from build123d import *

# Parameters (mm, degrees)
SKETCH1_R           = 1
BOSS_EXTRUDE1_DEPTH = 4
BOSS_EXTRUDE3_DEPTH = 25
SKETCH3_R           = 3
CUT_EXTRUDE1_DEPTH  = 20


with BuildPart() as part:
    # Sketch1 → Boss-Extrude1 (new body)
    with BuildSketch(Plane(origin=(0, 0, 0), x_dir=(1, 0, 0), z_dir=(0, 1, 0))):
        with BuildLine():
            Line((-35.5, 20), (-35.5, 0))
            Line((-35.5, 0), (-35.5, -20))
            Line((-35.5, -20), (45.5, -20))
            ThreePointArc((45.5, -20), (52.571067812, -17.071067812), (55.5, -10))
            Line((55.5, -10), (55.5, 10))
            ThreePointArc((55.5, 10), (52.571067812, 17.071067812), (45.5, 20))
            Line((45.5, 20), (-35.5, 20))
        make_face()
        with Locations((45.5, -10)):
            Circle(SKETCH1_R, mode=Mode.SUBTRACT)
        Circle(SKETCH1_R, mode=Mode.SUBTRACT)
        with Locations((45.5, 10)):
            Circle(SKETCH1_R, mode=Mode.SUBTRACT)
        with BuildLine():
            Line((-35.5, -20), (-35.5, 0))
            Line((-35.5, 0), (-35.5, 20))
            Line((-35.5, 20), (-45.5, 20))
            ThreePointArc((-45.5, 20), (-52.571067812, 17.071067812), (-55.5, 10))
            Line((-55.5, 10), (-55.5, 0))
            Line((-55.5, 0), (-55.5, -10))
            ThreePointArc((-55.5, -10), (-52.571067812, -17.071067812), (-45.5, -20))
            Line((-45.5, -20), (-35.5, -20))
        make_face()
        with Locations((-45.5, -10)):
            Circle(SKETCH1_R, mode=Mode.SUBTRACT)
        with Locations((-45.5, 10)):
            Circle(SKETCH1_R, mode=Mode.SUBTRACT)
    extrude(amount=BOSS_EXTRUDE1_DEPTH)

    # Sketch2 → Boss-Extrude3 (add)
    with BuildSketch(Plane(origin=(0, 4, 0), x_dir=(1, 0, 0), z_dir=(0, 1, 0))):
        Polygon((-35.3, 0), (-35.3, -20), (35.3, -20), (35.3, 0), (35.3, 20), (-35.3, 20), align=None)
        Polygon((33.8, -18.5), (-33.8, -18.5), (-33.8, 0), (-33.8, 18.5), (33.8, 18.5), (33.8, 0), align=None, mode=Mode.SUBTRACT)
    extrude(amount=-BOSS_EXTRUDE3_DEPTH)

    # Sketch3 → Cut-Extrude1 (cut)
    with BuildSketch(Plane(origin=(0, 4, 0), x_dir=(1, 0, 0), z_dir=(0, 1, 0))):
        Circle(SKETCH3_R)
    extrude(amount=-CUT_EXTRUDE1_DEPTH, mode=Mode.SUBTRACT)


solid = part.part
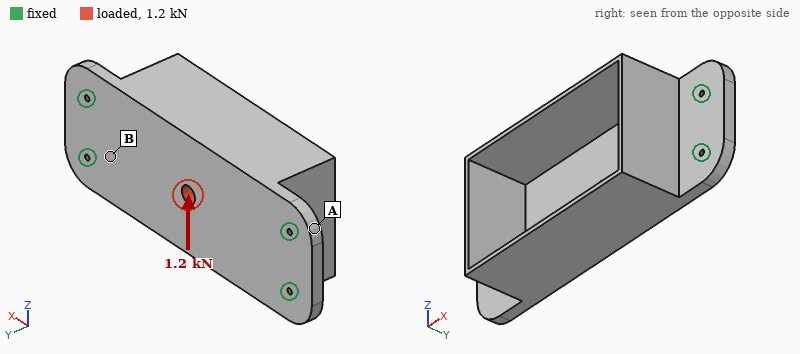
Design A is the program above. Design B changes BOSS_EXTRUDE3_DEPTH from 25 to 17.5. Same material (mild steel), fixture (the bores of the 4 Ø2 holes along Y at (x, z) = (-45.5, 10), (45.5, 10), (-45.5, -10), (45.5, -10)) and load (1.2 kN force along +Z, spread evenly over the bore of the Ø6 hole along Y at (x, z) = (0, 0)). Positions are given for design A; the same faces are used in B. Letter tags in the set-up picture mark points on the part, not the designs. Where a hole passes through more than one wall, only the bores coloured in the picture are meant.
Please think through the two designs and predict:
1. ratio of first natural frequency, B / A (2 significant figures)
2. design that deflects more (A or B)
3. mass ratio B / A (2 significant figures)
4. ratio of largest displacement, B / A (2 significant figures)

1.1
B
0.90
1.2
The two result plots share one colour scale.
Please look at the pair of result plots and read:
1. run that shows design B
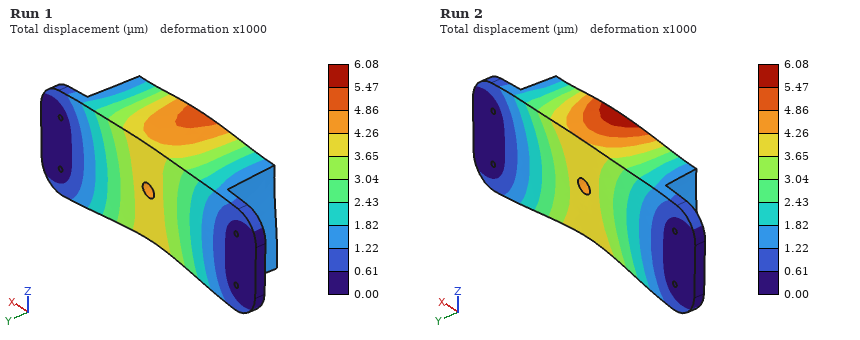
Run 2
